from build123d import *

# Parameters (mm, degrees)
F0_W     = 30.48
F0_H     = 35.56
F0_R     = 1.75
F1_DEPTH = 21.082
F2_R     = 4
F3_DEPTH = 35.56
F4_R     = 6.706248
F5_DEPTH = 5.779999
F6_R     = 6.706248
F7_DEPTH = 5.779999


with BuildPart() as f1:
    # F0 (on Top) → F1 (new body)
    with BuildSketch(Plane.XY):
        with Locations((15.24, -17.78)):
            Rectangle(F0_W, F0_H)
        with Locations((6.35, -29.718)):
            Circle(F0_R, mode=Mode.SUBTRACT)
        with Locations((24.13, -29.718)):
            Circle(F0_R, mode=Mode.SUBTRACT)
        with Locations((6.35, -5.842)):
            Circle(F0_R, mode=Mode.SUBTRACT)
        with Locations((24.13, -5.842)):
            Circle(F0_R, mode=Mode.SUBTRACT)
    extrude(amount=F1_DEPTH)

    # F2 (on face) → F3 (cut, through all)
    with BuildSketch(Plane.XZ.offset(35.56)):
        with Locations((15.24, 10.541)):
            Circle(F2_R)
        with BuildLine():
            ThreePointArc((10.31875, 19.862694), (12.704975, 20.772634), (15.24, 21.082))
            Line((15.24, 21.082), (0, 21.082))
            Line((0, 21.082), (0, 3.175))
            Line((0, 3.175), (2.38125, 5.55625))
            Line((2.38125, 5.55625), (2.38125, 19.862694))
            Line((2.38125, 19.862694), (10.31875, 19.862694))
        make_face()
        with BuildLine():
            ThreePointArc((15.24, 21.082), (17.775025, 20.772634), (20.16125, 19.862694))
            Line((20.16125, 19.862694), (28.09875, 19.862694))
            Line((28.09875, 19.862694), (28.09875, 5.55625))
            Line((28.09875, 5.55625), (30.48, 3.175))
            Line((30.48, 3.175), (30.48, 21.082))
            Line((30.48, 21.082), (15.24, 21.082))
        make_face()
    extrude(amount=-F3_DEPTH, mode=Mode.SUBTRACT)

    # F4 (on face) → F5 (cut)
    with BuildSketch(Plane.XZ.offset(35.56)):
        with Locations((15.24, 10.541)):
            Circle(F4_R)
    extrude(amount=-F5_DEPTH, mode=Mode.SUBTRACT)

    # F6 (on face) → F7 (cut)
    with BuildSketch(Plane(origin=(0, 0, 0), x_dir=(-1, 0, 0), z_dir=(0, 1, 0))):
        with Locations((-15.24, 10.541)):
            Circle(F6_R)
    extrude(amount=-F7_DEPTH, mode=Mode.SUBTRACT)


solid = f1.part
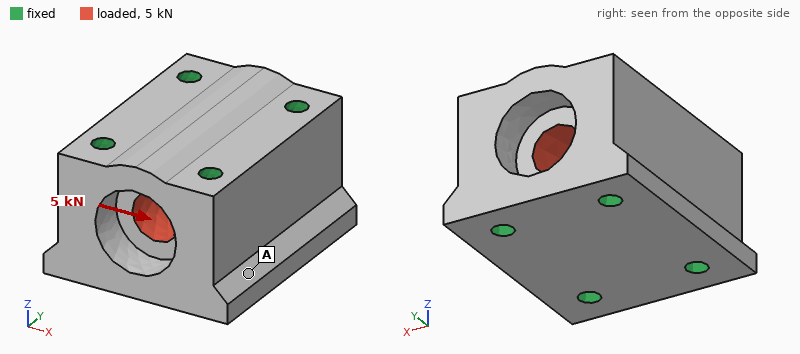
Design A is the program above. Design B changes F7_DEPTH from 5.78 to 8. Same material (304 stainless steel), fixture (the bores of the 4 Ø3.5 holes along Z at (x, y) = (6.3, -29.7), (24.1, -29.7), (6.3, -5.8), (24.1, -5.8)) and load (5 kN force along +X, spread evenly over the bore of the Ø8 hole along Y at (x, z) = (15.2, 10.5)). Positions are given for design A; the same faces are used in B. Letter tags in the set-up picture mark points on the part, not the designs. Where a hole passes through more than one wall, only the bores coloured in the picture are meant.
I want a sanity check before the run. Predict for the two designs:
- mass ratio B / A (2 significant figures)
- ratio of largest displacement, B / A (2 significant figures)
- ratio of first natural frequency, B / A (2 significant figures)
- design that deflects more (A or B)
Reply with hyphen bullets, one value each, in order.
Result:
- 0.99
- 1.1
- 0.99
- B
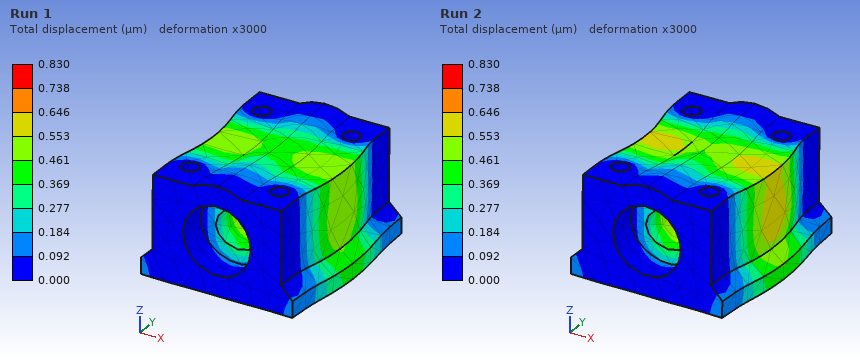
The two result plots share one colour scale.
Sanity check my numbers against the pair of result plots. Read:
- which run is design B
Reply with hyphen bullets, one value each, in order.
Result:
- Run 2
